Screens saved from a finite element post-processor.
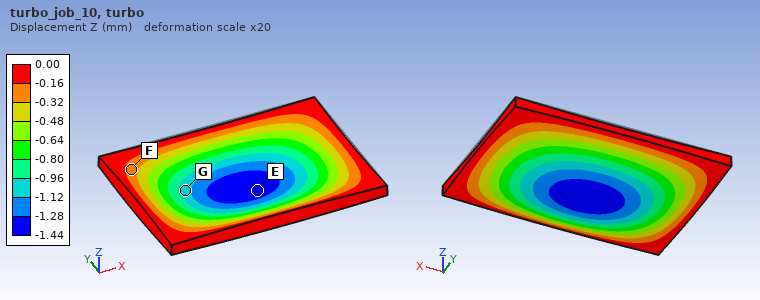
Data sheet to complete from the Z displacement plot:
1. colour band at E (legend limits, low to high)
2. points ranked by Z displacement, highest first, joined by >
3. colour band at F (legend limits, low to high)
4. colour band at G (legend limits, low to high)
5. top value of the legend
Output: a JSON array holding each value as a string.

["-1.44 to -1.28 mm", "F > G > E", "-0.32 to -0.16 mm", "-1.12 to -0.96 mm", "0.00 mm"]
